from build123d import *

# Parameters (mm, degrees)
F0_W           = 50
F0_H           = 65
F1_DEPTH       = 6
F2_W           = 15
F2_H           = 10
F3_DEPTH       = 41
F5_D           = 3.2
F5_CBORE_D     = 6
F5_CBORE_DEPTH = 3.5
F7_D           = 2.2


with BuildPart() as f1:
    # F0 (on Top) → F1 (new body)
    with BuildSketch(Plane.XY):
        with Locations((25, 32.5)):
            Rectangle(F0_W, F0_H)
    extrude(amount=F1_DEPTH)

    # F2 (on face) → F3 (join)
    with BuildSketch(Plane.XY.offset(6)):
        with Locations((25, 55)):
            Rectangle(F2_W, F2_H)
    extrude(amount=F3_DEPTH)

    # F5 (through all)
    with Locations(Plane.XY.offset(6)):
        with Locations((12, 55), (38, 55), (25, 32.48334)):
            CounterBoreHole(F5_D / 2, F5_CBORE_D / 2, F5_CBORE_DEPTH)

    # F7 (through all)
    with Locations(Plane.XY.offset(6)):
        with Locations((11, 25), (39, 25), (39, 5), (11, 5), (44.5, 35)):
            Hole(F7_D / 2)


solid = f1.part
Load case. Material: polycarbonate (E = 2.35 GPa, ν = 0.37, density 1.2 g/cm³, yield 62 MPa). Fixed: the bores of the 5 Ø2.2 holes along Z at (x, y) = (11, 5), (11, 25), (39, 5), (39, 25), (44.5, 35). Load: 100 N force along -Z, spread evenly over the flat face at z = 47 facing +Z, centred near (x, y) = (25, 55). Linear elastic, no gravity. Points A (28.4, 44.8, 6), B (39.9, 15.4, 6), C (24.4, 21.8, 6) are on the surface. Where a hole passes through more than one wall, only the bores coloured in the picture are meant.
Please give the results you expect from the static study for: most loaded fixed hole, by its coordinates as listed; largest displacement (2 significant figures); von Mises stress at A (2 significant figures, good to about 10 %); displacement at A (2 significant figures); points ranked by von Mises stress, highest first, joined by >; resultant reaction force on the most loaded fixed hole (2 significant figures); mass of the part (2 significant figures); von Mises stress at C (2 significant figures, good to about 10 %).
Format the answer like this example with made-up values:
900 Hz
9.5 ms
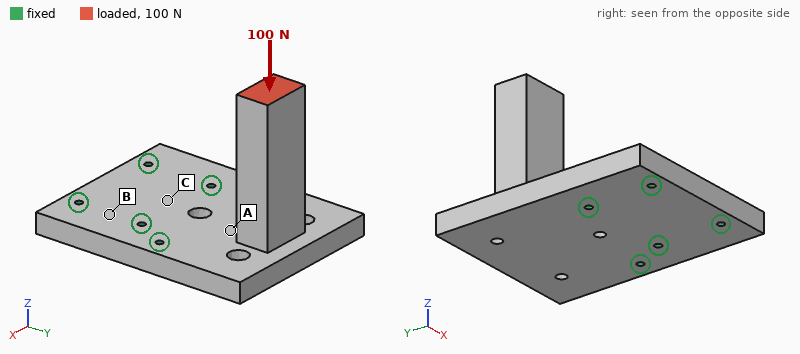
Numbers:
(44.5, 35)
0.96 mm
3.7 MPa
0.19 mm
A > C > B
88 N
30 g
2.2 MPa
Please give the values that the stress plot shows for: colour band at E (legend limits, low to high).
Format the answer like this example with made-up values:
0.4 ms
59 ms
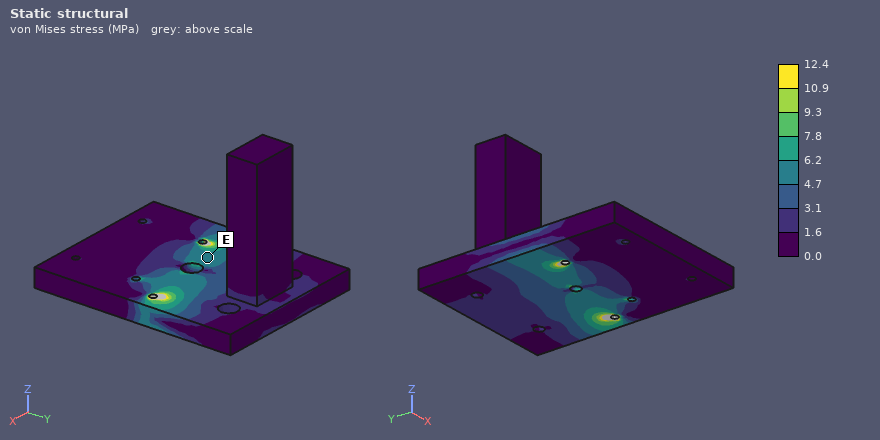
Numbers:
4.7 to 6.2 MPa
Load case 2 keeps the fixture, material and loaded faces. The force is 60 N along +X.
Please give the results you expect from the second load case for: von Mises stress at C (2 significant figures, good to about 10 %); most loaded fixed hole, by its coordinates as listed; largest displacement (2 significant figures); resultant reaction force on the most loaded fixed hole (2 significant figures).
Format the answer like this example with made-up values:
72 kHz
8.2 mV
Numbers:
1.4 MPa
(11, 25)
0.99 mm
100 N
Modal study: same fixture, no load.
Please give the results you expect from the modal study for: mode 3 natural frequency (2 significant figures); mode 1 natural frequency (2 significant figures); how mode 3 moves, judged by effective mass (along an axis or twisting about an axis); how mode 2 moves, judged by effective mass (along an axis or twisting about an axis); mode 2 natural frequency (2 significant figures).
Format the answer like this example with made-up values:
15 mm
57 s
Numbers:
1300 Hz
450 Hz
along Z
along X
780 Hz
